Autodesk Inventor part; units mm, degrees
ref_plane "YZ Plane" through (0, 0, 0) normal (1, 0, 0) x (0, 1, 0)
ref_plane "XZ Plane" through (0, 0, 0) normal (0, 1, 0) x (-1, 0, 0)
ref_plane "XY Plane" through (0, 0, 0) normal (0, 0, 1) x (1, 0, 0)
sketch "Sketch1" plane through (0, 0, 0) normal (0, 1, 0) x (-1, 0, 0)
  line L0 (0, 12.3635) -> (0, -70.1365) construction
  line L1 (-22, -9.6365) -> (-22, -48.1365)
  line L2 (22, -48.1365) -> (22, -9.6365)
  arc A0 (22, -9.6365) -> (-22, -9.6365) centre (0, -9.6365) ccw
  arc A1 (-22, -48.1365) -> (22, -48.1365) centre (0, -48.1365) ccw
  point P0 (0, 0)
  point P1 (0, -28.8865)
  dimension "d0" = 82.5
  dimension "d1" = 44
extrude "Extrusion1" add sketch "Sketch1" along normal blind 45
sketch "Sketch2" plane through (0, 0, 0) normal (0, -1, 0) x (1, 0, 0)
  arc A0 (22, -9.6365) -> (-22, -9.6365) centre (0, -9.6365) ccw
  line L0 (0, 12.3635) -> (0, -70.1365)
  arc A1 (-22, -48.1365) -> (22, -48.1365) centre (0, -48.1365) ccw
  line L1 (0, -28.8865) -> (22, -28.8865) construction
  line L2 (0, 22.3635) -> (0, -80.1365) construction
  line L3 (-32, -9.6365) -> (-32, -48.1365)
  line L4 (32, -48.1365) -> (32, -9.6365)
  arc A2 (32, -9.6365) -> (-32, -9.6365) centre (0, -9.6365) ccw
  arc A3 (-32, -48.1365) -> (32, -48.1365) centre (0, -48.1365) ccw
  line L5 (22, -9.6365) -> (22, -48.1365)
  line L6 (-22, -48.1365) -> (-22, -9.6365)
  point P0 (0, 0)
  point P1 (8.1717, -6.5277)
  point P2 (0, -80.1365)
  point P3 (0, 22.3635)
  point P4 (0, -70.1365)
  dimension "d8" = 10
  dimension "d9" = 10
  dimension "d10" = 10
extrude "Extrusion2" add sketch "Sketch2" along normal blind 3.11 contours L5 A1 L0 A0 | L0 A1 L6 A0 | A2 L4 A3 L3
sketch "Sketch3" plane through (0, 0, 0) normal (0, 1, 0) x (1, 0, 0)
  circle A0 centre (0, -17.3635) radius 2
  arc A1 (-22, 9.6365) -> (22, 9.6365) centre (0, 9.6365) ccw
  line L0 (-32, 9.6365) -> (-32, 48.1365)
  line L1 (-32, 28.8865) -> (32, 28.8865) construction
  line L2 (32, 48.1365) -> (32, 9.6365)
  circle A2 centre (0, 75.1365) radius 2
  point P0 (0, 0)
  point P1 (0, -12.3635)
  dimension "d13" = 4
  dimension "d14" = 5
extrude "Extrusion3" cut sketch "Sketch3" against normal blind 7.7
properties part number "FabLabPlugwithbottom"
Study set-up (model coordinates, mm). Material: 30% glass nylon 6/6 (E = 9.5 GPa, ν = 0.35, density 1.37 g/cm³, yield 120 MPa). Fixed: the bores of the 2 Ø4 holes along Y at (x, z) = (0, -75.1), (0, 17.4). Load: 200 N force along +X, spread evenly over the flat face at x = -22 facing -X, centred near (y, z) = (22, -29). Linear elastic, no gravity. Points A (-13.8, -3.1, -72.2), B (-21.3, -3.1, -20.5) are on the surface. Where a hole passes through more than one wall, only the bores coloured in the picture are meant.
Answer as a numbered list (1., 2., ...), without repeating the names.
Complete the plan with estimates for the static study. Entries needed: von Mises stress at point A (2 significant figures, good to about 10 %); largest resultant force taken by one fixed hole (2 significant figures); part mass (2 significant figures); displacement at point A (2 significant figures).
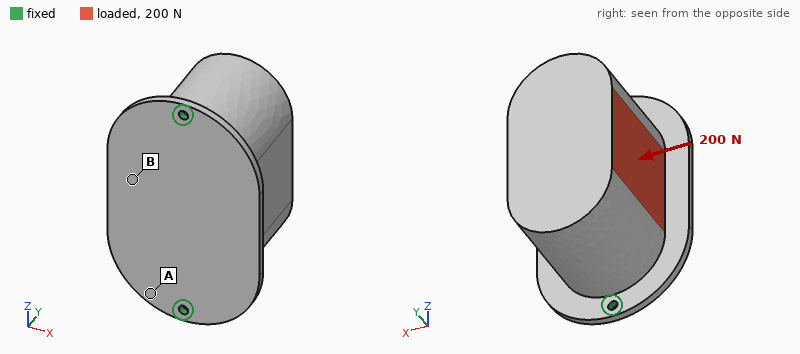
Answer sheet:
1. 8.3 MPa
2. 100 N
3. 220 g
4. 0.18 mm
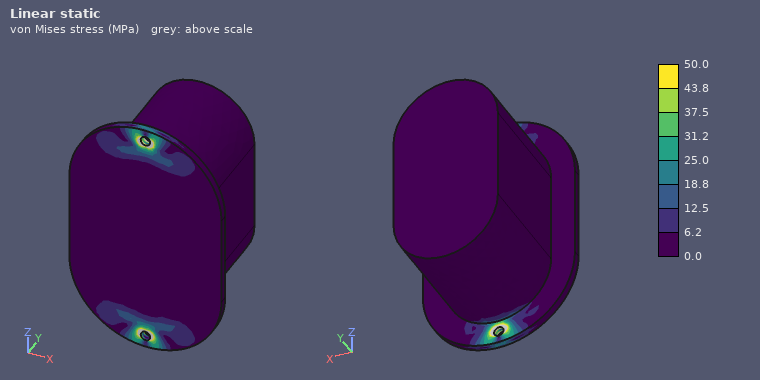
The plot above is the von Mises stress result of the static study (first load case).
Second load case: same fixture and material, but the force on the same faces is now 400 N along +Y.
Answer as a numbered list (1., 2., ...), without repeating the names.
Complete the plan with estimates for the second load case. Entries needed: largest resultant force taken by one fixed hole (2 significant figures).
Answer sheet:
1. 230 N
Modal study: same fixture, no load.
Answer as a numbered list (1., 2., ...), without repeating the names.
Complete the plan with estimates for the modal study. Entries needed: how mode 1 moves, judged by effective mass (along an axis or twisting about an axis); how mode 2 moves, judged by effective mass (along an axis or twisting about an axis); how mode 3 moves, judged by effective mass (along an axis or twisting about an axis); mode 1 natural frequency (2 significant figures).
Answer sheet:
1. along X
2. along Y
3. along Z
4. 210 Hz
